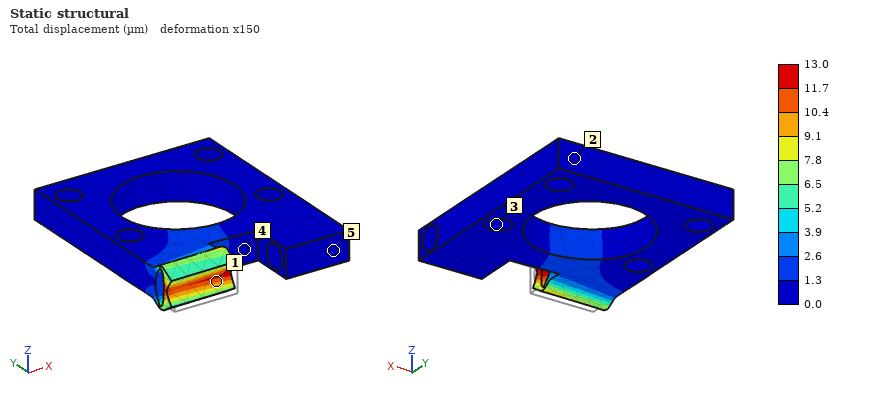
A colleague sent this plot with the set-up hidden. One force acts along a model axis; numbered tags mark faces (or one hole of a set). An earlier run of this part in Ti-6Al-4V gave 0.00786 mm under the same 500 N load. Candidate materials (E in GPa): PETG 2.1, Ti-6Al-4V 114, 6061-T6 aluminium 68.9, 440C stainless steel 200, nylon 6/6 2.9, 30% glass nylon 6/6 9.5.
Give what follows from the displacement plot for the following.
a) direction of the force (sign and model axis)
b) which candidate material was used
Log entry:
+Y
6061-T6 aluminium
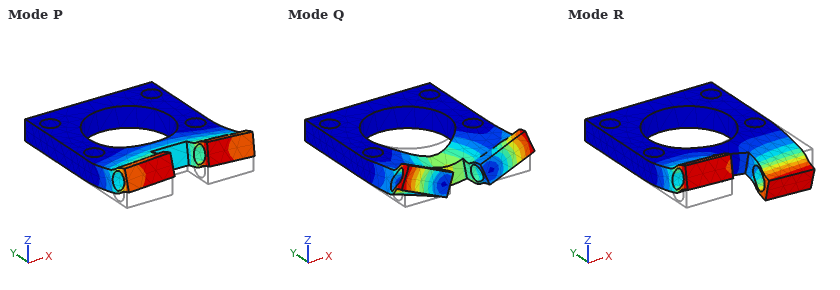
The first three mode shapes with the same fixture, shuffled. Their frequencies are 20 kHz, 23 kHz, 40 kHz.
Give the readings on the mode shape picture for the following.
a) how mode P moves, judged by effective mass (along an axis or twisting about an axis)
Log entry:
along Z
